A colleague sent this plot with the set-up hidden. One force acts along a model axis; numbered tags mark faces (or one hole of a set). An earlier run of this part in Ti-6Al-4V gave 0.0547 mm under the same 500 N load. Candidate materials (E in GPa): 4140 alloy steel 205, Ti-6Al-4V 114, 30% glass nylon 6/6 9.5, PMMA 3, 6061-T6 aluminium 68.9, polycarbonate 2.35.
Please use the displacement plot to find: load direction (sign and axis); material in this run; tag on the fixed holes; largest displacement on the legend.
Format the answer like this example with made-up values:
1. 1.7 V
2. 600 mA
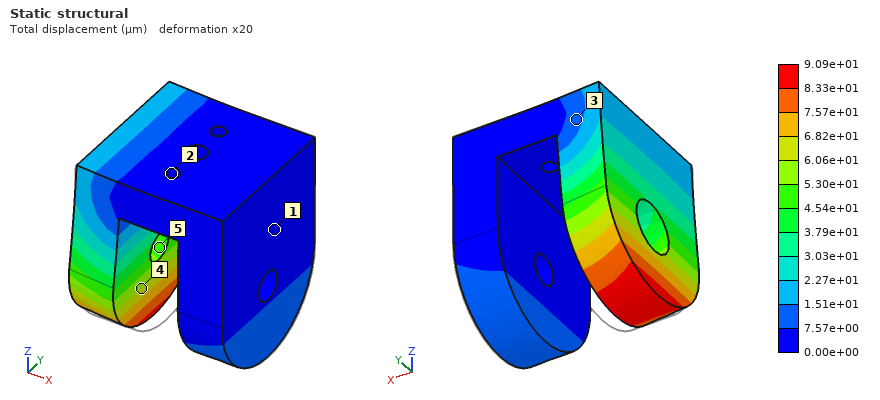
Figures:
1. -X
2. 6061-T6 aluminium
3. 2
4. 9.09e+01 µm
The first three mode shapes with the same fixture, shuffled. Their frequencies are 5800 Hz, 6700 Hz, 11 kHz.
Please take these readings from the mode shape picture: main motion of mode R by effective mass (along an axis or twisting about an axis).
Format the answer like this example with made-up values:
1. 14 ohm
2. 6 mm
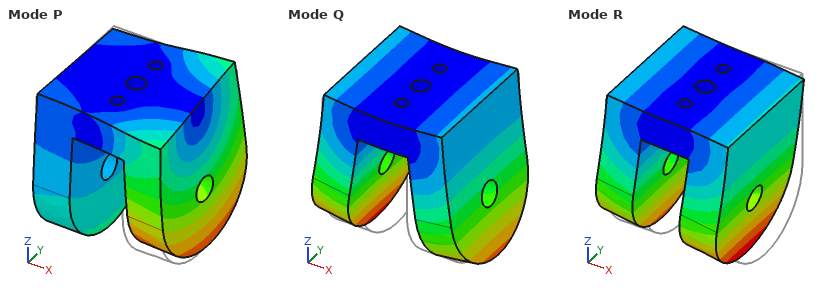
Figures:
1. along X
